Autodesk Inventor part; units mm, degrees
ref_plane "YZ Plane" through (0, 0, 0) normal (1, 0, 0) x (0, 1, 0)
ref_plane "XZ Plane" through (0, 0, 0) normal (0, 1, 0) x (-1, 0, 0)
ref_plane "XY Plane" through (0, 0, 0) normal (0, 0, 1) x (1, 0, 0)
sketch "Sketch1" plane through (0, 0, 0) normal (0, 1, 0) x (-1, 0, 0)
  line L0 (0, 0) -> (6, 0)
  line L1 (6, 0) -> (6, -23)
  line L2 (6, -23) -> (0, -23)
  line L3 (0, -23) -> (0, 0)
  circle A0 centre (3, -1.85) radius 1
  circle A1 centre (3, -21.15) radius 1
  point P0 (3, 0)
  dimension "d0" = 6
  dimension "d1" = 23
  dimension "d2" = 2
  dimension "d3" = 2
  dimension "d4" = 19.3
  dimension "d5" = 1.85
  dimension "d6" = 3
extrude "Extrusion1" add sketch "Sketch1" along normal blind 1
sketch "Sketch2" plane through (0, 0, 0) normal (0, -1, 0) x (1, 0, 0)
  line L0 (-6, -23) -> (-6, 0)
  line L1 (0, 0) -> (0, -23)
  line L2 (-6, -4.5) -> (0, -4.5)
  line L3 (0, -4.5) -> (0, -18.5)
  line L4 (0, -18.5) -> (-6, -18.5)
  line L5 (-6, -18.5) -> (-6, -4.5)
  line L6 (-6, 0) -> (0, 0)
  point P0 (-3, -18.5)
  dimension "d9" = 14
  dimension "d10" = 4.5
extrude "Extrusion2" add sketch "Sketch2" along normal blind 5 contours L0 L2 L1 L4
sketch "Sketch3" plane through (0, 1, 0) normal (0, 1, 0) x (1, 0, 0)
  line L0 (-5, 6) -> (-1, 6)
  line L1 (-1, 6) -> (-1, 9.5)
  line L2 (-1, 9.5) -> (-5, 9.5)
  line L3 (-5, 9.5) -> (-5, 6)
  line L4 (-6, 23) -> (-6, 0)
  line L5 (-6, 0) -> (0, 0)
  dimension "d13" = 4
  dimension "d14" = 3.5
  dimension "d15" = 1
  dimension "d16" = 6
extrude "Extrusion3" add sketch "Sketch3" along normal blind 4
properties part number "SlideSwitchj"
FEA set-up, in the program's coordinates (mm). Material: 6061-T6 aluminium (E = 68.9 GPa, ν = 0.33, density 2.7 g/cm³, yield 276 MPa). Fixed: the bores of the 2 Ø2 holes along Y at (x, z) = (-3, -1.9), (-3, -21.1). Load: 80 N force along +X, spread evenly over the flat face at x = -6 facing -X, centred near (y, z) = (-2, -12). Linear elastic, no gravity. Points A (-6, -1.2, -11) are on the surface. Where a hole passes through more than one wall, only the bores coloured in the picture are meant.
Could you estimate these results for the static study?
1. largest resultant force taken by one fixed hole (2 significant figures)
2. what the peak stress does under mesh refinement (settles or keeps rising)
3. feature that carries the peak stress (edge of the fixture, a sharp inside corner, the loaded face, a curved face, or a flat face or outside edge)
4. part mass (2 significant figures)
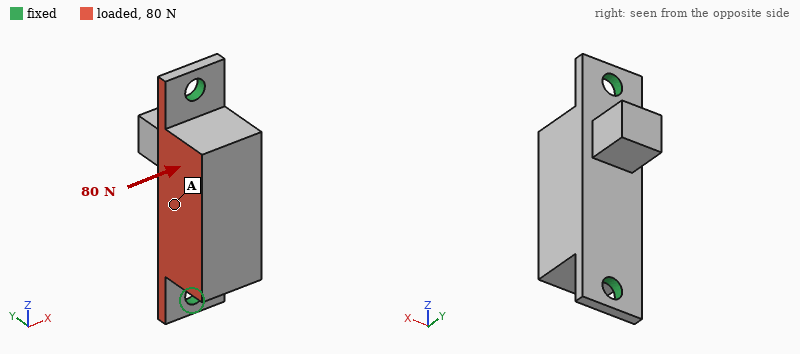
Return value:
40 N
keeps rising
edge of the fixture
1.6 g
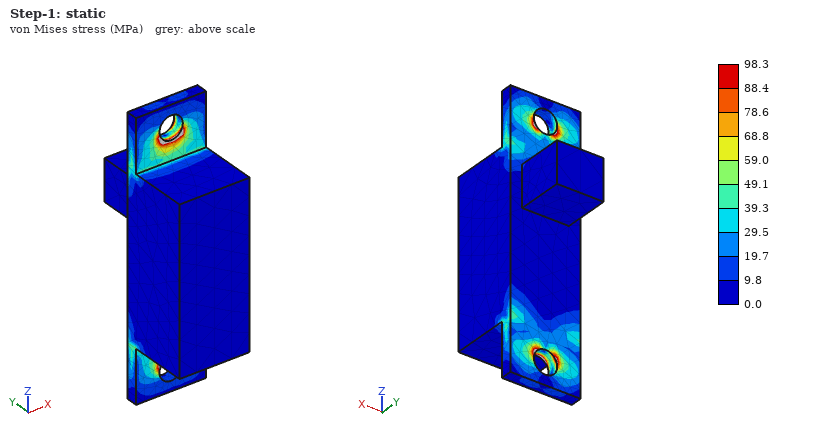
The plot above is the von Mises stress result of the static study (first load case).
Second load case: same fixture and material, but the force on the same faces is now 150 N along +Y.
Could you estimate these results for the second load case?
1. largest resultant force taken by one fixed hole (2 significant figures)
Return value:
87 N
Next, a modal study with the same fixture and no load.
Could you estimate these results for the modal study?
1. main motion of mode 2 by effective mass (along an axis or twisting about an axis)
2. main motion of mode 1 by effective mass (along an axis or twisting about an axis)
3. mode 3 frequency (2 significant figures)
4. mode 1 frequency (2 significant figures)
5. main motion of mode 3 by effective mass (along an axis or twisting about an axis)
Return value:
along Y
along X
33 kHz
9500 Hz
along X
